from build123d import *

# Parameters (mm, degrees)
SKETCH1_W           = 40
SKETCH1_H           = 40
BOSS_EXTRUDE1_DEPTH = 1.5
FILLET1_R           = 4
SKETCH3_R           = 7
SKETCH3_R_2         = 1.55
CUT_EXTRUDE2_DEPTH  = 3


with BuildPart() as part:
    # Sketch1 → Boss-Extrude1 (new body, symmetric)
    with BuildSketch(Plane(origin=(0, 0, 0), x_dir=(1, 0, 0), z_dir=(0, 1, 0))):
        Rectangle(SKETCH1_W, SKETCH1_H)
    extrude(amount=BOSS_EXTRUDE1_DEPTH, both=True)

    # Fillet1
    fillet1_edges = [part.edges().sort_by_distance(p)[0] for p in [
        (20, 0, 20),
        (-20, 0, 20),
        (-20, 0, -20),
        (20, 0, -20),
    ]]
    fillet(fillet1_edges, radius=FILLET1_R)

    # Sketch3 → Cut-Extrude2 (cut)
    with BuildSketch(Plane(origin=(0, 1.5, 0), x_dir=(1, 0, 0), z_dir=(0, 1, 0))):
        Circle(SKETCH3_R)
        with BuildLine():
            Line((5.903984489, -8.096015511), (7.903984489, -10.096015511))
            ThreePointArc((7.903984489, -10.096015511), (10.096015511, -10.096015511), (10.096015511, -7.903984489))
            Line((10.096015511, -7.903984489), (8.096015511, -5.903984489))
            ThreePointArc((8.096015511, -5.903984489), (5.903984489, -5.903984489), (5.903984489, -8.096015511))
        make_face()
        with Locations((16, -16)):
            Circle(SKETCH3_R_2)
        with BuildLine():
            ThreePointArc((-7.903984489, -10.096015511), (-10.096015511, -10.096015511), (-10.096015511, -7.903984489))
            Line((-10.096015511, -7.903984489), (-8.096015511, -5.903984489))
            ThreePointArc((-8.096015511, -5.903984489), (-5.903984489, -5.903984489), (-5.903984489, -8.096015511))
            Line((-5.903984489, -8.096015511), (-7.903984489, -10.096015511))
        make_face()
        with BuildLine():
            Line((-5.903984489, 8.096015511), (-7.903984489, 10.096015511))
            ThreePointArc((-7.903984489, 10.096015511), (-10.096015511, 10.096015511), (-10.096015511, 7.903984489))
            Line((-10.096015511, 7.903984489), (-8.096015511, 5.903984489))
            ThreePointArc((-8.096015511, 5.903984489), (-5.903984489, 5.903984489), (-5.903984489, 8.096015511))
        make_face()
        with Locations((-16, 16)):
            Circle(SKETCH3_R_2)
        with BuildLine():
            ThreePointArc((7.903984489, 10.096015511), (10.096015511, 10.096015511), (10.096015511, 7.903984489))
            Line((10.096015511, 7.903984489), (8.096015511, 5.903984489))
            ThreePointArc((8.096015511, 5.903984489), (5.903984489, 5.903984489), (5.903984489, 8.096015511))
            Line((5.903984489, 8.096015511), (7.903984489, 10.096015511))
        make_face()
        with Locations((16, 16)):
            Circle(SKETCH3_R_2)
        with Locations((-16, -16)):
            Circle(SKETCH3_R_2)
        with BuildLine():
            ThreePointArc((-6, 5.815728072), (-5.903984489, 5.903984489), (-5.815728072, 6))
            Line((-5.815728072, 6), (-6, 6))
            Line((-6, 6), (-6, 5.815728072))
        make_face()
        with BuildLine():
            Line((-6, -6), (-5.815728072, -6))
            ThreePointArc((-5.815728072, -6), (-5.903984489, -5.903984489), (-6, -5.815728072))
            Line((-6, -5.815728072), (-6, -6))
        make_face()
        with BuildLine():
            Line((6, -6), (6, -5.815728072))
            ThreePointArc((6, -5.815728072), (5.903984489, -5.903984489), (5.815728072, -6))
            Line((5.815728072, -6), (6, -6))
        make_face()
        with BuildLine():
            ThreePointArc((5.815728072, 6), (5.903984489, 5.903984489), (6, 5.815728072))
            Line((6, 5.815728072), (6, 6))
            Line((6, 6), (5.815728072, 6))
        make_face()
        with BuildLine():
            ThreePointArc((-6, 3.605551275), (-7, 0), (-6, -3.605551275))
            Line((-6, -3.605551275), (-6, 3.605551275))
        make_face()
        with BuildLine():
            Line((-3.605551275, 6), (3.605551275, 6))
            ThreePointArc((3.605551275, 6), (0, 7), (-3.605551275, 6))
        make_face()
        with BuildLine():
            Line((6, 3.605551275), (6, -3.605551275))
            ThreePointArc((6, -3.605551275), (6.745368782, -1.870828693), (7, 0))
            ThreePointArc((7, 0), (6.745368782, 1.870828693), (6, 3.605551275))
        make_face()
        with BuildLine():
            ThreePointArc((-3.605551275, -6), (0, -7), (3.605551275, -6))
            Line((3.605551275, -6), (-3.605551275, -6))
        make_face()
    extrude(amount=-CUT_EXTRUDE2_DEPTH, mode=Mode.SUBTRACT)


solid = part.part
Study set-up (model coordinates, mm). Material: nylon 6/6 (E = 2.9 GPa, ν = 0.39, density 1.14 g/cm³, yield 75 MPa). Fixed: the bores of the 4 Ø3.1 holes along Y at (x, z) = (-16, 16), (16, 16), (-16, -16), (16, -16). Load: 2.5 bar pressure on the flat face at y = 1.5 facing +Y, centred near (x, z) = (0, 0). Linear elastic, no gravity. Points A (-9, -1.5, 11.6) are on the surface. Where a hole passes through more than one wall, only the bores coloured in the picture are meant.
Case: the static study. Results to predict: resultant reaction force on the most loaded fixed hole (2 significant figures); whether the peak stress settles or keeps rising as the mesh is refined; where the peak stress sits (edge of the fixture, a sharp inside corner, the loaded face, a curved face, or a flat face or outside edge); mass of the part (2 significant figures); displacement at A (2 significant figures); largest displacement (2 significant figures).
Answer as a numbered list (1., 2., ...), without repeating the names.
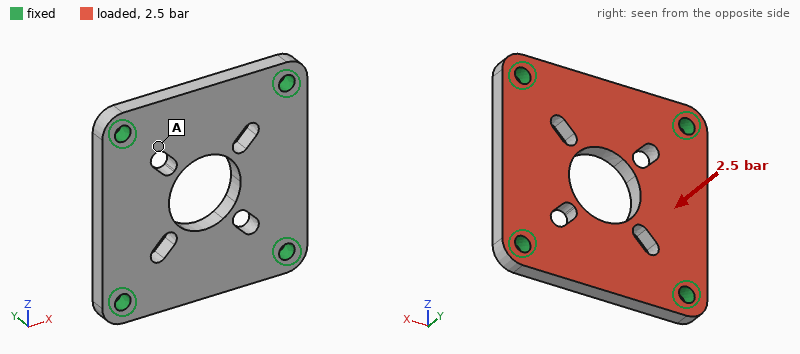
1. 84 N
2. keeps rising
3. edge of the fixture
4. 4.6 g
5. 0.10 mm
6. 0.22 mm
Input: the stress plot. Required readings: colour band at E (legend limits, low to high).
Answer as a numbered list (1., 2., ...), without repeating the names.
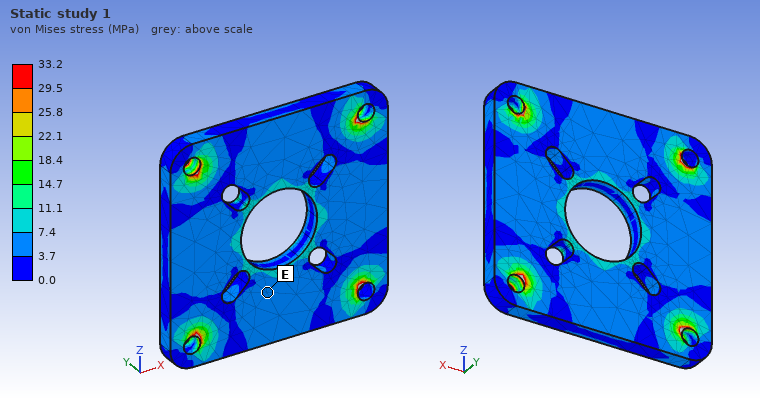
1. 3.7 to 7.4 MPa
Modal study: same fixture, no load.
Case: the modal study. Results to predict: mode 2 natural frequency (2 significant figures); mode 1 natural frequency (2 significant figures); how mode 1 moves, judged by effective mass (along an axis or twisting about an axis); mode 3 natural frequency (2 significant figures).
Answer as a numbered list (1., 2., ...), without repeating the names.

1. 5200 Hz
2. 3600 Hz
3. along Y
4. 5200 Hz
